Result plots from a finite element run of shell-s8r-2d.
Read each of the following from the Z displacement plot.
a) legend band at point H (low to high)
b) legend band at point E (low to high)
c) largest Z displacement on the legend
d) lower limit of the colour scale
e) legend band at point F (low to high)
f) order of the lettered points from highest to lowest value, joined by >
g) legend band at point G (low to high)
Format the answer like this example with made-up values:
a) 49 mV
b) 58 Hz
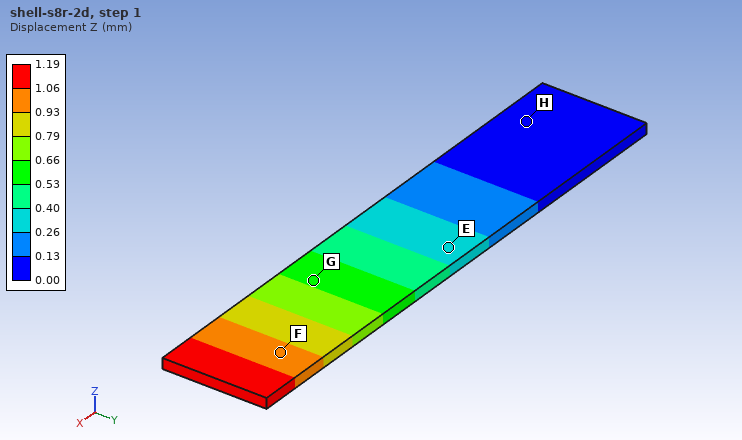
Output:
a) 0.00 to 0.13 mm
b) 0.26 to 0.40 mm
c) 1.19 mm
d) 0.00 mm
e) 0.93 to 1.06 mm
f) F > G > E > H
g) 0.53 to 0.66 mm
